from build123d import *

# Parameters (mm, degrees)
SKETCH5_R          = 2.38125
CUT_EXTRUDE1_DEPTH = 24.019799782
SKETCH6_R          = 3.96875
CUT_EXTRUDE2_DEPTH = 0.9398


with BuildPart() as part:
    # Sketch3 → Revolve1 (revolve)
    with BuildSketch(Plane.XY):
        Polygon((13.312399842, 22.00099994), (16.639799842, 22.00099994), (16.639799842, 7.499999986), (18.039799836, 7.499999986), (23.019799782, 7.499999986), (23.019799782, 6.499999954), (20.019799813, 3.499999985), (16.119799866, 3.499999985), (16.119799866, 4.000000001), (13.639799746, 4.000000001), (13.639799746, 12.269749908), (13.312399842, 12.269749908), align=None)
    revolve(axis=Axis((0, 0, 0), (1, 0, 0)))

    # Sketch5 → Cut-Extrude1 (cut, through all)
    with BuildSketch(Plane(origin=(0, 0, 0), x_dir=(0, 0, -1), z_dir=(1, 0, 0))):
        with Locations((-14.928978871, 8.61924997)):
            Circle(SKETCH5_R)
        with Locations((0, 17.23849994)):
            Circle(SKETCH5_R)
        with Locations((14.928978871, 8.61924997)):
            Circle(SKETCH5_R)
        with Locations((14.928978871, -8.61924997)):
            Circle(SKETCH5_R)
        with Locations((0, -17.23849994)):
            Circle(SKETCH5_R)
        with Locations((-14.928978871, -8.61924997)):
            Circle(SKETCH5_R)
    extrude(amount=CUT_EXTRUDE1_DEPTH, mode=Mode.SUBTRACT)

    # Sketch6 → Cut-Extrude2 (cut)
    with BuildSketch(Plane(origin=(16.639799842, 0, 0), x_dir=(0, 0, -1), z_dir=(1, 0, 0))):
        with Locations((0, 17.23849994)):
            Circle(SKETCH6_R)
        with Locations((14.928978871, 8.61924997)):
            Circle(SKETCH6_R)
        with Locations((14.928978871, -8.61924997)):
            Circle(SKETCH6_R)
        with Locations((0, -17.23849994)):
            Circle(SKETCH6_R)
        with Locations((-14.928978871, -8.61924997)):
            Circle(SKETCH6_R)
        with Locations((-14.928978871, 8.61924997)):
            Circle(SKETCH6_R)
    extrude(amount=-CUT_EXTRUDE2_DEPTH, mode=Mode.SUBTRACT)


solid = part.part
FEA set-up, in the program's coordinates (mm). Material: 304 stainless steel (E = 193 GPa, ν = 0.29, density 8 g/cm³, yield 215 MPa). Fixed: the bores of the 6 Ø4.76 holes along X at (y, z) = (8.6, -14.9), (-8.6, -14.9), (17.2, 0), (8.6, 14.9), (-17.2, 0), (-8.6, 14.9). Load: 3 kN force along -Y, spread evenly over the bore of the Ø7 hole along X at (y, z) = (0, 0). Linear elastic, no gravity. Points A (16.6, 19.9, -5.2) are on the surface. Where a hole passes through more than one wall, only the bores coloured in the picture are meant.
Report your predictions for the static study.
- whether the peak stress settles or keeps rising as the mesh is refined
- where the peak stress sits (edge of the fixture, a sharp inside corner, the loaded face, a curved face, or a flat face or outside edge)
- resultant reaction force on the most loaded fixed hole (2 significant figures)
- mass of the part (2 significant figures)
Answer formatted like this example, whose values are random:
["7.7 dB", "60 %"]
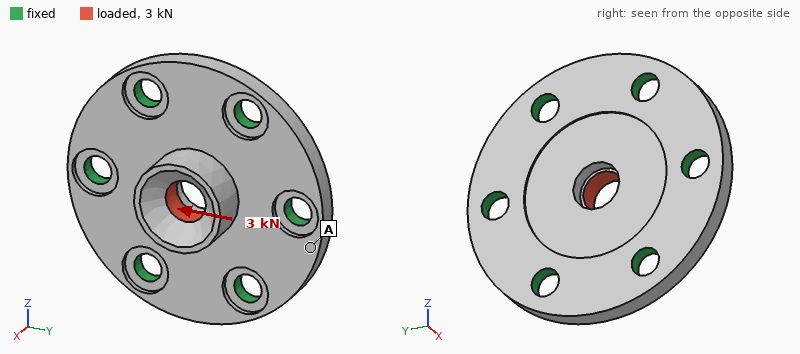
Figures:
["keeps rising", "edge of the fixture", "850 N", "40 g"]
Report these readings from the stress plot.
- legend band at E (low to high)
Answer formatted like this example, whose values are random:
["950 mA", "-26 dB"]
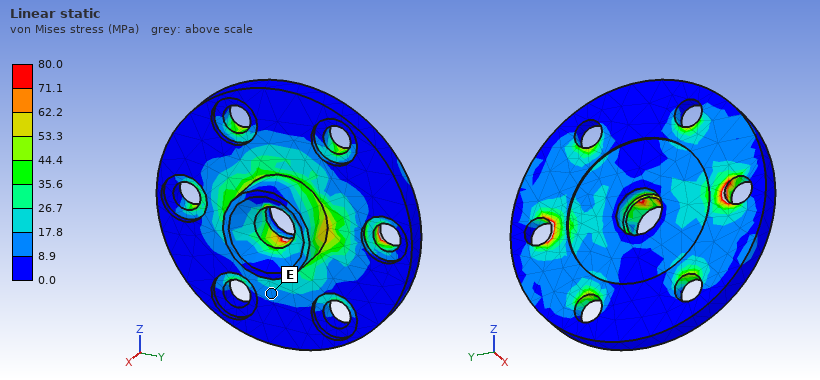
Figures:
["8.9 to 17.8 MPa"]
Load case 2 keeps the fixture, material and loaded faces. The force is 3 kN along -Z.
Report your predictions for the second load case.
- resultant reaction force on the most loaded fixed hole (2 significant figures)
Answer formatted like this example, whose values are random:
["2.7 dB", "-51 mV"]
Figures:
["740 N"]
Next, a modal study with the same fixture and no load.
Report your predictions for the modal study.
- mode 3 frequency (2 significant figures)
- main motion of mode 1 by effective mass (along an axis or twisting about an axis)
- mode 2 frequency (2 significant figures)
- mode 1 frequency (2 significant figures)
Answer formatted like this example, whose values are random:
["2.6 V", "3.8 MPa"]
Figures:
["33 kHz", "along X", "33 kHz", "23 kHz"]
